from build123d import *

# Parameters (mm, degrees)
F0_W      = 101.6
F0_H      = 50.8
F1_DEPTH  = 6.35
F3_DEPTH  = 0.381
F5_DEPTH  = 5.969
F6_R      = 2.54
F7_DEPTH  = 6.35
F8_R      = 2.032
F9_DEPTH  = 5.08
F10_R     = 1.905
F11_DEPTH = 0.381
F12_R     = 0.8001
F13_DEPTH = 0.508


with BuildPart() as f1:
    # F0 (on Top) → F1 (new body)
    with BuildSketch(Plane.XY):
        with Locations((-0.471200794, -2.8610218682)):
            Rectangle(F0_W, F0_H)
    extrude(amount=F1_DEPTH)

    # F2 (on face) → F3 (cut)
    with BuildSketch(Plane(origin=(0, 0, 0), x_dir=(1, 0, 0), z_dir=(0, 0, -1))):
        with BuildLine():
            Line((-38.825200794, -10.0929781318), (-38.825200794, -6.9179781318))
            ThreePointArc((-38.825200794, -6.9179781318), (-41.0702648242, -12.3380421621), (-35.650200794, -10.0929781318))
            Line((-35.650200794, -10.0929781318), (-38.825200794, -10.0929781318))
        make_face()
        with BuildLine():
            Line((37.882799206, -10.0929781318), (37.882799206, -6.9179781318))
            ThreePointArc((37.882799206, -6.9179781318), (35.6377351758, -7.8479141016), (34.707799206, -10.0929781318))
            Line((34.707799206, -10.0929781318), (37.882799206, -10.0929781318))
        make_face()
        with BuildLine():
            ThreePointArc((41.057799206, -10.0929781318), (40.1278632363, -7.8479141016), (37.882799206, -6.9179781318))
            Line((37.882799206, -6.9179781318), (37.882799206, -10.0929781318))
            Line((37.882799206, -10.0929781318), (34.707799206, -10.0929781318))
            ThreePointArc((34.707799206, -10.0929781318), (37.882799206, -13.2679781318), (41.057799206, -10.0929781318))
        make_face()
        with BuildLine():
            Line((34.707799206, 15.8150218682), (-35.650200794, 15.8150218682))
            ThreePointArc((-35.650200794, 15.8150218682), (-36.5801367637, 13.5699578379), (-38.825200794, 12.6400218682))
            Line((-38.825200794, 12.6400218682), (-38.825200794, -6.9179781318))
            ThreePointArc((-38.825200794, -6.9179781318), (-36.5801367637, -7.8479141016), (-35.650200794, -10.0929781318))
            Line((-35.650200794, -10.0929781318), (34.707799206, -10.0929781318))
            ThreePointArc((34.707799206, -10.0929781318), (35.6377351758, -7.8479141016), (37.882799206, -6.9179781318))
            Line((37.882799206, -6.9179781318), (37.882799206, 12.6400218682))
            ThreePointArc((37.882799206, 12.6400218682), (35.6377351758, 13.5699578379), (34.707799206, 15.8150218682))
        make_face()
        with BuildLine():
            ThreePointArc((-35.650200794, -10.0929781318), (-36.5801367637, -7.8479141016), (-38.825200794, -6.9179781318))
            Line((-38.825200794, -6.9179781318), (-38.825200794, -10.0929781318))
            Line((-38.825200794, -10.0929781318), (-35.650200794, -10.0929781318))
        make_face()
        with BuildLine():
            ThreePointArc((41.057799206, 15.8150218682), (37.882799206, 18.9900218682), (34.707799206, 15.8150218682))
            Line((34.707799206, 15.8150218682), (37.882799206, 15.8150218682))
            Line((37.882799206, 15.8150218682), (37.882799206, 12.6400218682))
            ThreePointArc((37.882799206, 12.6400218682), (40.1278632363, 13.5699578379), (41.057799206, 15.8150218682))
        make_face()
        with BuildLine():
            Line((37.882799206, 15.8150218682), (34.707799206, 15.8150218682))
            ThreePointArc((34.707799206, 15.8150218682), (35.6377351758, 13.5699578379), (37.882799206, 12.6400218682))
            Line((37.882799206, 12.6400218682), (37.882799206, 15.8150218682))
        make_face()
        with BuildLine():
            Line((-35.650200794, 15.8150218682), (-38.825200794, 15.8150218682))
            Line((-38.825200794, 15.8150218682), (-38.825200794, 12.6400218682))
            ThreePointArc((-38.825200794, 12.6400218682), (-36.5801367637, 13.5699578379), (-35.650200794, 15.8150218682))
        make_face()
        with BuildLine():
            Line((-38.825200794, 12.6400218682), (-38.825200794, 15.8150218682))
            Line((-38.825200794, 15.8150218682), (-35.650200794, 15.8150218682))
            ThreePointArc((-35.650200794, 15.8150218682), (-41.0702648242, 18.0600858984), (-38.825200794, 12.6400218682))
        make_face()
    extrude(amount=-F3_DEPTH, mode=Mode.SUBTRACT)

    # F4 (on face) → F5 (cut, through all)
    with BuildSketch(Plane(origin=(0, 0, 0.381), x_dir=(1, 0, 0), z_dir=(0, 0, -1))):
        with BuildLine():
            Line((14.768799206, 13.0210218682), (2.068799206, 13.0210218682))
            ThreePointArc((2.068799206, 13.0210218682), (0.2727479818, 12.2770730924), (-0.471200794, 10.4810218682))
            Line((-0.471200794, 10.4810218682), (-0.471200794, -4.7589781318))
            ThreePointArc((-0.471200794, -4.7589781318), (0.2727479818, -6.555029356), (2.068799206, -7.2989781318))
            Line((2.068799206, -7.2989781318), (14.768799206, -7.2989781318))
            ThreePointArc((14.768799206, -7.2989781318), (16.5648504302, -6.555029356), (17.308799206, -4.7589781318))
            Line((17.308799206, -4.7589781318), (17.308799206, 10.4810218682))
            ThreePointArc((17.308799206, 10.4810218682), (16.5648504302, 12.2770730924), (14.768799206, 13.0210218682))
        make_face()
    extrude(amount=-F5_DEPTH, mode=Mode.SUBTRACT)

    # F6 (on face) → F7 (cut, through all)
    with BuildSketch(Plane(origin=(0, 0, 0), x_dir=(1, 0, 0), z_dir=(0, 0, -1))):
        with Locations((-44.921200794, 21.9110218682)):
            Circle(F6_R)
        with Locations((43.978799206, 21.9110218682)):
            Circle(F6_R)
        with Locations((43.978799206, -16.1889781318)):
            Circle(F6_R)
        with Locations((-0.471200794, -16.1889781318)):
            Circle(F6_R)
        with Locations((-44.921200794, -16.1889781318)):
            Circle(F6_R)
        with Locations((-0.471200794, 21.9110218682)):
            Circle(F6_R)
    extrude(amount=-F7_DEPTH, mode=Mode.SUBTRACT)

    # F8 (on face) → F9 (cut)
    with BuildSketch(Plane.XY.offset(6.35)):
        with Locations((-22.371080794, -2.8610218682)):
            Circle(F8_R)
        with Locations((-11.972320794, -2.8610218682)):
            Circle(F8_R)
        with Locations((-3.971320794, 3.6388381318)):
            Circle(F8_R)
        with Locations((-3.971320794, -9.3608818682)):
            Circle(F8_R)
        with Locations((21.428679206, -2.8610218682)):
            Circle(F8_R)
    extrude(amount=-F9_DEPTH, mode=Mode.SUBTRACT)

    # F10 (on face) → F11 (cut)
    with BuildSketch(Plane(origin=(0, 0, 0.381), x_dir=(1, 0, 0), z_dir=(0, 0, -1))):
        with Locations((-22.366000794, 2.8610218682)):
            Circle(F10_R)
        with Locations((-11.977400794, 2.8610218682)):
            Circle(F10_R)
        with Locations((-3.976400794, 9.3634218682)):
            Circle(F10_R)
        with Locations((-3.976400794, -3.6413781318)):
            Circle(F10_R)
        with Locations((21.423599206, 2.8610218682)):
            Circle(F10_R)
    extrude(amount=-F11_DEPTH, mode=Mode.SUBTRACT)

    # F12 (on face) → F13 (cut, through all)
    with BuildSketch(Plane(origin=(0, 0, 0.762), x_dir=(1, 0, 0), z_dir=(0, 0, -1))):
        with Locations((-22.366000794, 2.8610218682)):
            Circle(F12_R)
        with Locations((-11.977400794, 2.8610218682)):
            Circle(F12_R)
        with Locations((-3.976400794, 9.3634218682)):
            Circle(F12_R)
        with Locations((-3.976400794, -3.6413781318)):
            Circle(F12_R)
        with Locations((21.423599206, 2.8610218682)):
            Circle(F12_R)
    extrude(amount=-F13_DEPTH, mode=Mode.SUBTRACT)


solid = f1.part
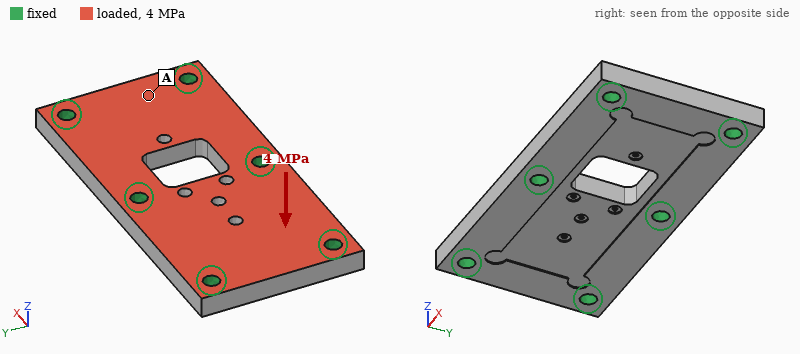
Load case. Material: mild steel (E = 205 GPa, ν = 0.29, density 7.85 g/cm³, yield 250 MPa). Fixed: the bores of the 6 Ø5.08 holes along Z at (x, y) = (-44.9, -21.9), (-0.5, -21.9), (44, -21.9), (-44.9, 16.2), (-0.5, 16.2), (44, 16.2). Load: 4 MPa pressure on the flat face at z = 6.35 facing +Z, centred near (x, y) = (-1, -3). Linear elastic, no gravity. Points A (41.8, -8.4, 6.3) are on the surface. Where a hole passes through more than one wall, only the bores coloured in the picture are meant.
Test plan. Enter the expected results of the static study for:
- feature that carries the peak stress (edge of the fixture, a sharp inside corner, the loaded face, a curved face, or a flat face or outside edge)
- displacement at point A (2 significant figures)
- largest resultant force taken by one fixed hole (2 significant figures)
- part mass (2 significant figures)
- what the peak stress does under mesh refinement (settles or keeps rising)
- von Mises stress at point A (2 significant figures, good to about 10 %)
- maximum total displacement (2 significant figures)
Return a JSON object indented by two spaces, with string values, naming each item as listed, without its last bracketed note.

{
  "feature that carries the peak stress": "edge of the fixture",
  "displacement at point A": "8.1 µm",
  "largest resultant force taken by one fixed hole": "3.8 kN",
  "part mass": "230 g",
  "what the peak stress does under mesh refinement": "keeps rising",
  "von Mises stress at point A": "34 MPa",
  "maximum total displacement": "22 µm"
}
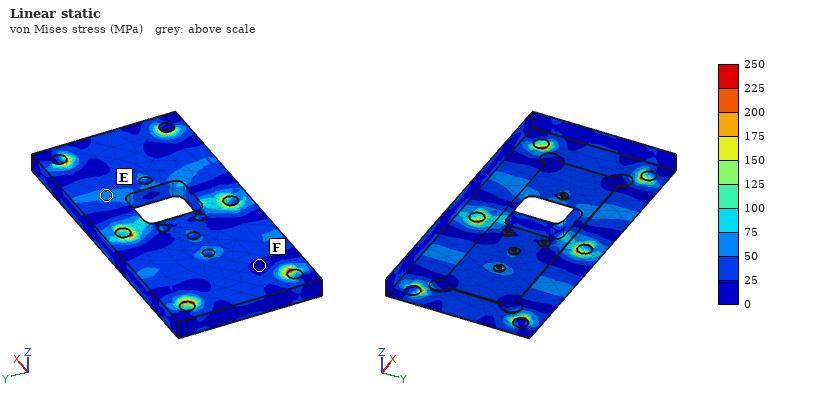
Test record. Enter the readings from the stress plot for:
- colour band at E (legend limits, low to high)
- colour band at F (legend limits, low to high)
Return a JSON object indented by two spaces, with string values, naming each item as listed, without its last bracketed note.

{
  "colour band at E": "50 to 75 MPa",
  "colour band at F": "0 to 25 MPa"
}
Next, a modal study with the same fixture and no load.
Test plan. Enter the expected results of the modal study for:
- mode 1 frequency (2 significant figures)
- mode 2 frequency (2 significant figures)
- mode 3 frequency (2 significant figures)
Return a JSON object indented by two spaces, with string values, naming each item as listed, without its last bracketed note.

{
  "mode 1 frequency": "12 kHz",
  "mode 2 frequency": "13 kHz",
  "mode 3 frequency": "17 kHz"
}
